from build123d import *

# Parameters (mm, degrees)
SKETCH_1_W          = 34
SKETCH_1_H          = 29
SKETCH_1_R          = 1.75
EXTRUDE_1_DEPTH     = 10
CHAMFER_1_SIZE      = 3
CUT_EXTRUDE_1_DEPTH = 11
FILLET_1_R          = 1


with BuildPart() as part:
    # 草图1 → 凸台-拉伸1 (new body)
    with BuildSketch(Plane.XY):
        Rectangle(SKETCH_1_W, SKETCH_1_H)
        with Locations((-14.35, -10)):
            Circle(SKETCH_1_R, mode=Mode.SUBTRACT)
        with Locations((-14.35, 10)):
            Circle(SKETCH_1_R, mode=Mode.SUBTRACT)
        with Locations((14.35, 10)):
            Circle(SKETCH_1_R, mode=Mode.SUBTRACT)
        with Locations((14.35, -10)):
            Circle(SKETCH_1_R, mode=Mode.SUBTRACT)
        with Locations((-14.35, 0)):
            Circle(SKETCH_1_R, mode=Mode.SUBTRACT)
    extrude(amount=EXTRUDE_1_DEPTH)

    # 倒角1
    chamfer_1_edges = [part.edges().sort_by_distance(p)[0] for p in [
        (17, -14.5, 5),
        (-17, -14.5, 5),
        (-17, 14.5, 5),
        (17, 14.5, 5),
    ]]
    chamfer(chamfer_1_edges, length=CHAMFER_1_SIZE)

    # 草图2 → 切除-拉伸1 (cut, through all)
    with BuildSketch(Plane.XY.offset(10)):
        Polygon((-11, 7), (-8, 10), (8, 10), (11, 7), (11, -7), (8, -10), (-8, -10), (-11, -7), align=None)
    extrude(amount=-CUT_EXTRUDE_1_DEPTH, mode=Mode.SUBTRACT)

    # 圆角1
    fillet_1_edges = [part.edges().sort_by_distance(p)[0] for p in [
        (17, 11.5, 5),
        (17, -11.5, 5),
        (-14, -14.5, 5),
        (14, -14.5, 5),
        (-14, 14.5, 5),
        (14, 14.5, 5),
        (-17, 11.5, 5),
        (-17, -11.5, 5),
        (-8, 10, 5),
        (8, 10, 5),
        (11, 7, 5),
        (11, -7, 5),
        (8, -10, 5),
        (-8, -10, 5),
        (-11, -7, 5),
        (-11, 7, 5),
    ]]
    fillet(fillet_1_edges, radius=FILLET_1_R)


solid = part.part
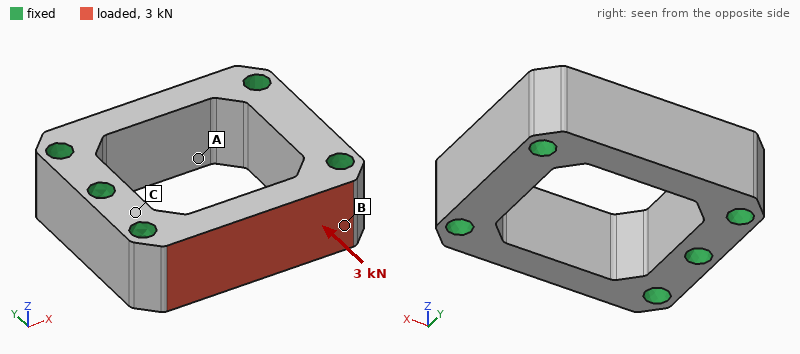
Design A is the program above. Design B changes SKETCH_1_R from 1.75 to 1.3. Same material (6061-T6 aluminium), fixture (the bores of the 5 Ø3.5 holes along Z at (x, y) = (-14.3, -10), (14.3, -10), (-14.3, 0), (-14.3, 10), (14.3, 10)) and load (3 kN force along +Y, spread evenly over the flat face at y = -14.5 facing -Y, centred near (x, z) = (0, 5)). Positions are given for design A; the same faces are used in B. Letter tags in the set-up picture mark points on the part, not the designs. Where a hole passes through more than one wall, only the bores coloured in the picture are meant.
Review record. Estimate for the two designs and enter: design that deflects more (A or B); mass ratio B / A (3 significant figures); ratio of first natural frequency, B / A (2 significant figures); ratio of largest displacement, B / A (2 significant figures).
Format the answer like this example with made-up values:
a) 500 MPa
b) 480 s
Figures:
a) B
b) 1.04
c) 0.93
d) 1.1
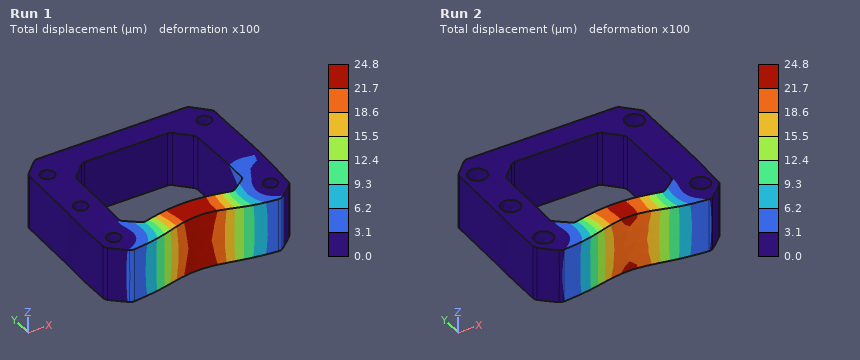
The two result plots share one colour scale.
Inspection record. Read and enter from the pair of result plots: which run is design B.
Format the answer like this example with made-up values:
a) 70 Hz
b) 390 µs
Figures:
a) Run 1
